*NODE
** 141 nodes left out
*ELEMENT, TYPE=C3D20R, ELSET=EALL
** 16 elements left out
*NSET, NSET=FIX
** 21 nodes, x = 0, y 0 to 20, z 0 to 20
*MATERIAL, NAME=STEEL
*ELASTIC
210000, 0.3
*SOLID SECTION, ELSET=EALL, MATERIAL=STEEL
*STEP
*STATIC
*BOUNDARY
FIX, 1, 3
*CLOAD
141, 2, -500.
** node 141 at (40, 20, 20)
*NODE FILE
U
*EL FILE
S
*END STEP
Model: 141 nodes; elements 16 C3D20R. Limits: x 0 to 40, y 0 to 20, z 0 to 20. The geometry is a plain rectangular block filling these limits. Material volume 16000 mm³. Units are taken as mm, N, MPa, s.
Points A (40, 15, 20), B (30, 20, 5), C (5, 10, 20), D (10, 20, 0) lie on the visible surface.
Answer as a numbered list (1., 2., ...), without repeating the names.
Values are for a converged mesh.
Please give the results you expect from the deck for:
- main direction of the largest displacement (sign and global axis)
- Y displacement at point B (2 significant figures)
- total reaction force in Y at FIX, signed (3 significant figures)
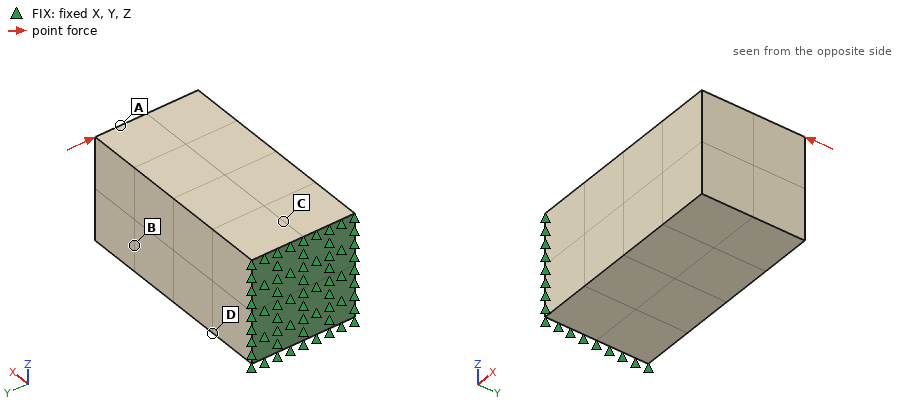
1. -Y
2. -0.0024 mm
3. 500 N
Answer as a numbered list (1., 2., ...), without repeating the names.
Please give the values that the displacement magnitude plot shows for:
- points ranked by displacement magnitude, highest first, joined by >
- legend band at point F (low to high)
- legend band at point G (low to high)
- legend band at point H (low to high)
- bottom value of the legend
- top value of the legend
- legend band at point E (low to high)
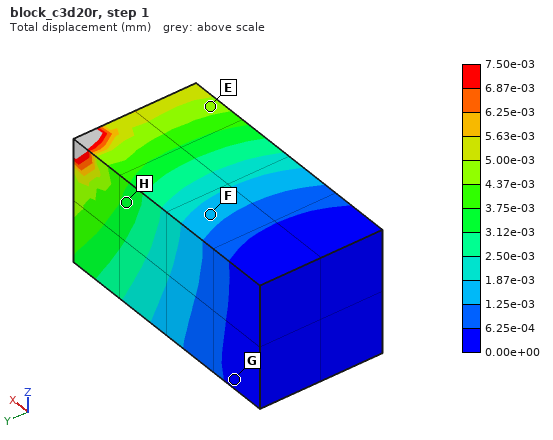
1. E > H > F > G
2. 1.25e-03 to 1.87e-03 mm
3. 0.00e+00 to 6.25e-04 mm
4. 3.12e-03 to 3.75e-03 mm
5. 0.00e+00 mm
6. 7.50e-03 mm
7. 4.37e-03 to 5.00e-03 mm
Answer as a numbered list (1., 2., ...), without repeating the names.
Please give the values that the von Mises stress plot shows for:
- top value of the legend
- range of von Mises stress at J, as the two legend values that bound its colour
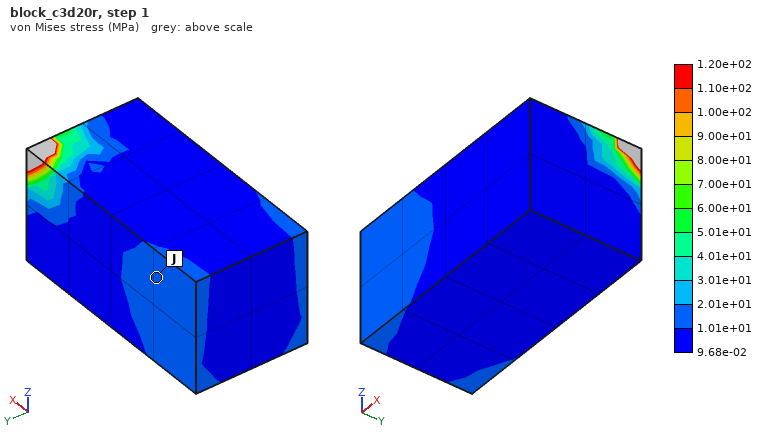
1. 1.20e+02 MPa
2. 1.01e+01 to 2.01e+01 MPa
